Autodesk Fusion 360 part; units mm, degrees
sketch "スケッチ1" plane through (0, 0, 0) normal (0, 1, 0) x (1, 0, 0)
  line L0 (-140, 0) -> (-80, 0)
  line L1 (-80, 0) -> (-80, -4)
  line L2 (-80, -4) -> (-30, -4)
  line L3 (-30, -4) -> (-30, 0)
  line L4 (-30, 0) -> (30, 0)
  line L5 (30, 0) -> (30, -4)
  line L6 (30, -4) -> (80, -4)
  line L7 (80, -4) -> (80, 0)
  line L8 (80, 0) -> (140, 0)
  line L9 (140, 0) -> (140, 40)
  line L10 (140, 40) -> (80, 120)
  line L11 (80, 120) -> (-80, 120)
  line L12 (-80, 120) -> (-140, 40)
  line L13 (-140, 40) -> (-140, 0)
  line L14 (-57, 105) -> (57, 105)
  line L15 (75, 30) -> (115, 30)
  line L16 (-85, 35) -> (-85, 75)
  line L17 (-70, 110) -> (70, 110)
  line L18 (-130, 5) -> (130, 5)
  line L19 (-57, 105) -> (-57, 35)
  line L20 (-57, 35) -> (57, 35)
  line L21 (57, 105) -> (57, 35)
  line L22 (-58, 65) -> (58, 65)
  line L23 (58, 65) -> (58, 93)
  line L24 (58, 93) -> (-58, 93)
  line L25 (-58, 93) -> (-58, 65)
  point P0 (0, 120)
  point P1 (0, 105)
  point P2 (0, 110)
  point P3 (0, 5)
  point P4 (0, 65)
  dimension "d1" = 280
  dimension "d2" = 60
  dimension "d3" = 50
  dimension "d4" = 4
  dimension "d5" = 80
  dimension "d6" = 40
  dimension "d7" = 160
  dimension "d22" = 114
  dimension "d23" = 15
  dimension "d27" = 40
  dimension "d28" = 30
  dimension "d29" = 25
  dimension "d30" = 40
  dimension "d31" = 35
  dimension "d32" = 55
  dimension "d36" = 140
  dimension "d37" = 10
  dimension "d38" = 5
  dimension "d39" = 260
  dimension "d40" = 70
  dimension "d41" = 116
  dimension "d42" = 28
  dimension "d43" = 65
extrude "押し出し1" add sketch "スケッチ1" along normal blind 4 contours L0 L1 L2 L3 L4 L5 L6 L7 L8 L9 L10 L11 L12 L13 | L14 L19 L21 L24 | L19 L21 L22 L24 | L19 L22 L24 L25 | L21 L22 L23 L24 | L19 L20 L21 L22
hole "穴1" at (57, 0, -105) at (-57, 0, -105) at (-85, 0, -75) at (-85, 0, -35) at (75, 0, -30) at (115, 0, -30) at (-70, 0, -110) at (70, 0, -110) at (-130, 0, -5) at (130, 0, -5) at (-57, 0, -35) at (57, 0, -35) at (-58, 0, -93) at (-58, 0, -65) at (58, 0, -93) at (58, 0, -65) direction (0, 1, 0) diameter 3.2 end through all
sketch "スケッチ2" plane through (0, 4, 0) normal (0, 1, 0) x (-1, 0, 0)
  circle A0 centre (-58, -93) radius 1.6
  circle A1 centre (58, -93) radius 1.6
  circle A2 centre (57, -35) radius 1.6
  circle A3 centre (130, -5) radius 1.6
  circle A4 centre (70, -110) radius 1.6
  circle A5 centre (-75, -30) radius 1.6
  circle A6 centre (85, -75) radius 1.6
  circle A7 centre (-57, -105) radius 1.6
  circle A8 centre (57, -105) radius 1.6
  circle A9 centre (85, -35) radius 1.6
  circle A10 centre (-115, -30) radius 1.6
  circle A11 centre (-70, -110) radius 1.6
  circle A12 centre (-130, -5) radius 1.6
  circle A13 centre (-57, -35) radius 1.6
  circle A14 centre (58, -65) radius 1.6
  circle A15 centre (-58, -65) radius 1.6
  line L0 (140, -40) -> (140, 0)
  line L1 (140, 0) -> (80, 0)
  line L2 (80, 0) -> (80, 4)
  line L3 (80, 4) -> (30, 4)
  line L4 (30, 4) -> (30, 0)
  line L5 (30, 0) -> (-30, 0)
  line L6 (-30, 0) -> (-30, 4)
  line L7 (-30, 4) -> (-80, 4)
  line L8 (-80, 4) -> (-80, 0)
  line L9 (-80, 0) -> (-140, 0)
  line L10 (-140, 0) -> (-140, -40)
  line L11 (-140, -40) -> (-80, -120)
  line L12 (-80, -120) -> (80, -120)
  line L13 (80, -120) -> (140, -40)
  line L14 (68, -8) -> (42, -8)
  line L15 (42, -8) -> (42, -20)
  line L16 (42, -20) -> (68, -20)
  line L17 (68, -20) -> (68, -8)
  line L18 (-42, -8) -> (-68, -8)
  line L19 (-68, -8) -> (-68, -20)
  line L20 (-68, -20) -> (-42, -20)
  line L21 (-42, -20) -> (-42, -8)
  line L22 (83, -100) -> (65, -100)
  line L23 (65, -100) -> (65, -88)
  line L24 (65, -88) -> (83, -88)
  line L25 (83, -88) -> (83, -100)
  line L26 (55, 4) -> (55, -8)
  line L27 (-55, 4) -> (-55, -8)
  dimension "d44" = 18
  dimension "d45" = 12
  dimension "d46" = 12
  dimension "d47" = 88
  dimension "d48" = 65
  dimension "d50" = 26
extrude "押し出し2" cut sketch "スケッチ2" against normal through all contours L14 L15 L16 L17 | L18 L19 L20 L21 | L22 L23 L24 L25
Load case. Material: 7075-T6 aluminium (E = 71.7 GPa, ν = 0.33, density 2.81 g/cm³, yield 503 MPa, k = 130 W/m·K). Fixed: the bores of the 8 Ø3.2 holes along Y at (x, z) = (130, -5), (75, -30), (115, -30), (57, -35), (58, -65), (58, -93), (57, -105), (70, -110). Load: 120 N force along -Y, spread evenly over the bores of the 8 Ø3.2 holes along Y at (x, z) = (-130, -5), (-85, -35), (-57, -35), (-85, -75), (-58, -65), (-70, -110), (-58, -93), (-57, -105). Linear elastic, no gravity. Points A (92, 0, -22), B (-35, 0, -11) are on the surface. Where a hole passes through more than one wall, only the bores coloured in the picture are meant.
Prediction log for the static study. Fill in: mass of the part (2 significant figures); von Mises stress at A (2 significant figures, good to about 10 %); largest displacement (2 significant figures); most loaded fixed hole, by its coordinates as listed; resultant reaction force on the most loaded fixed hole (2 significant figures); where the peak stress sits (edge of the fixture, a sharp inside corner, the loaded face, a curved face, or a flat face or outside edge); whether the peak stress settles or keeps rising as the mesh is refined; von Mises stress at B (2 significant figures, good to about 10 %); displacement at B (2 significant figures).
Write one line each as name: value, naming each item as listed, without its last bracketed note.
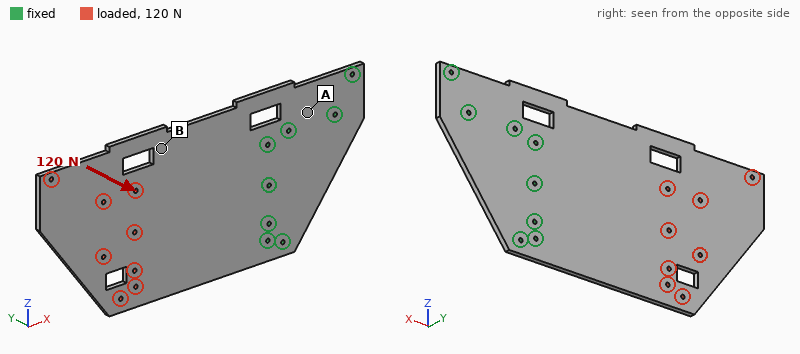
mass of the part: 320 g
von Mises stress at A: 4.4 MPa
largest displacement: 3.6 mm
most loaded fixed hole, by its coordinates as listed: (57, -35)
resultant reaction force on the most loaded fixed hole: 220 N
where the peak stress sits: edge of the fixture
whether the peak stress settles or keeps rising as the mesh is refined: keeps rising
von Mises stress at B: 14 MPa
displacement at B: 1.1 mm
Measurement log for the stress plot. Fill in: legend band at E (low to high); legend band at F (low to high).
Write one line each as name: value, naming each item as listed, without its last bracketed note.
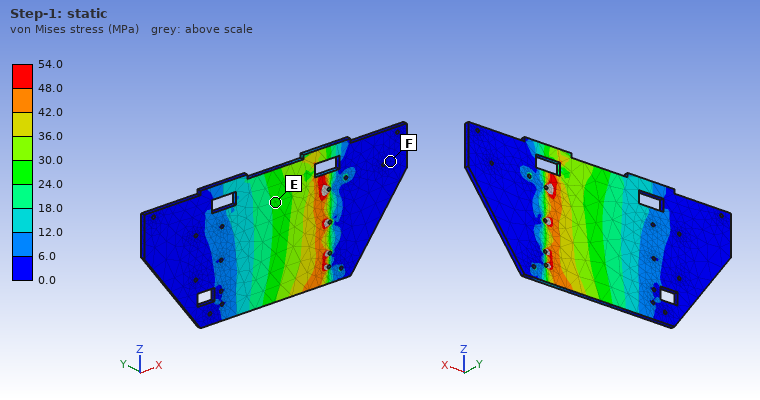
legend band at E: 24.0 to 30.0 MPa
legend band at F: 0.0 to 6.0 MPa
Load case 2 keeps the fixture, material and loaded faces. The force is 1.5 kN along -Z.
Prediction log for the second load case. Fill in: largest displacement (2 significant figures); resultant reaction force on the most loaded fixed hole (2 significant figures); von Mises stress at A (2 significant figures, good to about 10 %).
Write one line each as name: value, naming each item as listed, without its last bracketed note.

largest displacement: 96 µm
resultant reaction force on the most loaded fixed hole: 1.4 kN
von Mises stress at A: 4.4 MPa
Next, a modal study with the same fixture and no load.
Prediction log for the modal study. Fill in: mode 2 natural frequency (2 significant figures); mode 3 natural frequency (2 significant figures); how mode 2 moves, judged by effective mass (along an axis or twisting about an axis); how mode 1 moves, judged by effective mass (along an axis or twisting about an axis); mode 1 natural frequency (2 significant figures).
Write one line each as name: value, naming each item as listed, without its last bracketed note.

mode 2 natural frequency: 360 Hz
mode 3 natural frequency: 560 Hz
how mode 2 moves, judged by effective mass: twisting about X
how mode 1 moves, judged by effective mass: along Y
mode 1 natural frequency: 100 Hz
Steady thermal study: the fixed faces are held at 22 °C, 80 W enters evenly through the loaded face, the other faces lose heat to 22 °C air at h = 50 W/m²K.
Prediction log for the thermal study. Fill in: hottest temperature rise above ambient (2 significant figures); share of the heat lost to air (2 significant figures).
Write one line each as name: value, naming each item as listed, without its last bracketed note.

hottest temperature rise above ambient: 65 K
share of the heat lost to air: 82 %
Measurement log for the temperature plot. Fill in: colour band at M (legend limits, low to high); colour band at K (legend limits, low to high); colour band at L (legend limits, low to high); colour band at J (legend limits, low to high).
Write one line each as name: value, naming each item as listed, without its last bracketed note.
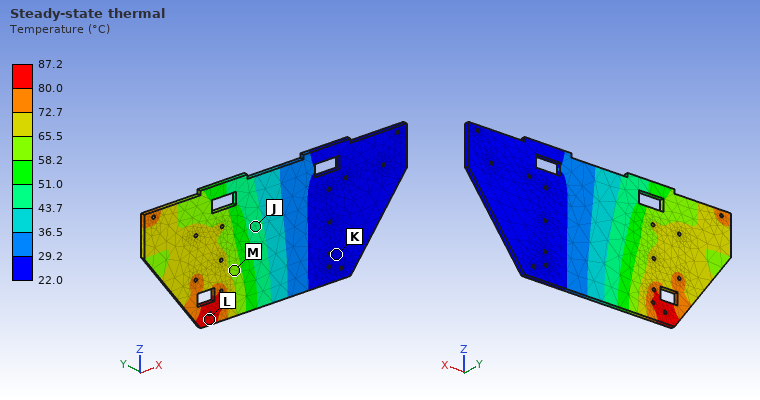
colour band at M: 58.2 to 65.5 °C
colour band at K: 22.0 to 29.2 °C
colour band at L: 80.0 to 87.2 °C
colour band at J: 43.7 to 51.0 °C
